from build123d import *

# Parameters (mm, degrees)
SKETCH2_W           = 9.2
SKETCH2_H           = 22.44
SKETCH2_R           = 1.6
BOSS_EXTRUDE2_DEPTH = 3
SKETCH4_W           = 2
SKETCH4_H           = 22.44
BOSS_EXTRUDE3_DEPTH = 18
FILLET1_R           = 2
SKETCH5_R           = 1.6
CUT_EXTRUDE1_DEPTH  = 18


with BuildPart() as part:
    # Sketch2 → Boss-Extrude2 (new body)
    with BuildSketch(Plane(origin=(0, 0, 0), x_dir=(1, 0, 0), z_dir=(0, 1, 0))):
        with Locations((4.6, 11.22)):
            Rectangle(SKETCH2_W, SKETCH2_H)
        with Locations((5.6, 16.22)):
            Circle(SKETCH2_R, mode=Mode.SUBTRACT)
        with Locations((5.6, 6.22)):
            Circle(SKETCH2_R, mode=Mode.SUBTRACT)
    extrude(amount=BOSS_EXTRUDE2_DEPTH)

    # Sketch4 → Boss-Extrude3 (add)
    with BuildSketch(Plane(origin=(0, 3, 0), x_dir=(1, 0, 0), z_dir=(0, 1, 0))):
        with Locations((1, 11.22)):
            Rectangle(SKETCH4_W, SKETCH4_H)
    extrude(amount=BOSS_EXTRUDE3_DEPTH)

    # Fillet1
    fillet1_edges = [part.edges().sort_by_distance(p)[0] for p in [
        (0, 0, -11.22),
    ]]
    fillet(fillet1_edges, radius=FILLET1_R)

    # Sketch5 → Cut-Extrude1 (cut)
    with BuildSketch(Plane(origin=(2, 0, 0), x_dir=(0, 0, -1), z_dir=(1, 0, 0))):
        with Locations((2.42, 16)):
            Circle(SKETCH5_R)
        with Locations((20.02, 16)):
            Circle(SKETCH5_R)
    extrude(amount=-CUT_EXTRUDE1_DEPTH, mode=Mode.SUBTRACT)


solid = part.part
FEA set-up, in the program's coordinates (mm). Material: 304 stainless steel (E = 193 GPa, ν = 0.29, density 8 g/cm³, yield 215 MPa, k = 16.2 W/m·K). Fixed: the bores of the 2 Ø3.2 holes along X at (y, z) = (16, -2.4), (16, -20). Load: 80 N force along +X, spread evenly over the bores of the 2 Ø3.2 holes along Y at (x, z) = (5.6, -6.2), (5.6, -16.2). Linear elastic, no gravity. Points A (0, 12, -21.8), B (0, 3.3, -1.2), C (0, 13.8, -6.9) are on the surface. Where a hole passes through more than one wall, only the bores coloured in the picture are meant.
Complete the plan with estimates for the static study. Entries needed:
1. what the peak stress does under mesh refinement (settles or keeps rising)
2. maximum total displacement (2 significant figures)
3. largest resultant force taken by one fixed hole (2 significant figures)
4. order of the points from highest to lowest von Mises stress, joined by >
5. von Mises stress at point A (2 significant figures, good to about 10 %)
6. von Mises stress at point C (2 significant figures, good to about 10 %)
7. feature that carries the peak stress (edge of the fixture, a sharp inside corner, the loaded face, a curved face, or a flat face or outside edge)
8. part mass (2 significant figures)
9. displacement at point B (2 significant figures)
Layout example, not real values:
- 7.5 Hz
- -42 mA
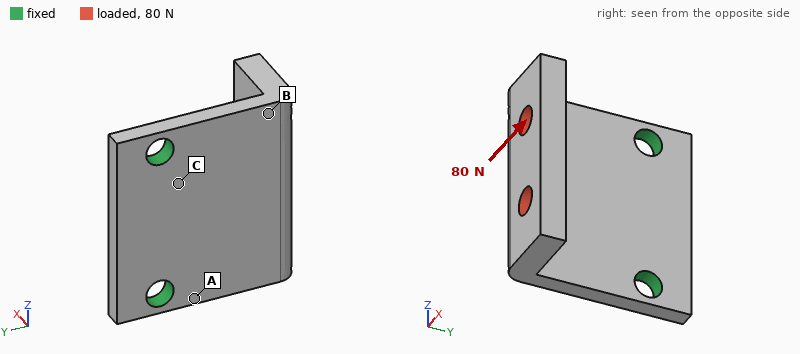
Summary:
- keeps rising
- 38 µm
- 40 N
- A > C > B
- 72 MPa
- 44 MPa
- edge of the fixture
- 11 g
- 22 µm
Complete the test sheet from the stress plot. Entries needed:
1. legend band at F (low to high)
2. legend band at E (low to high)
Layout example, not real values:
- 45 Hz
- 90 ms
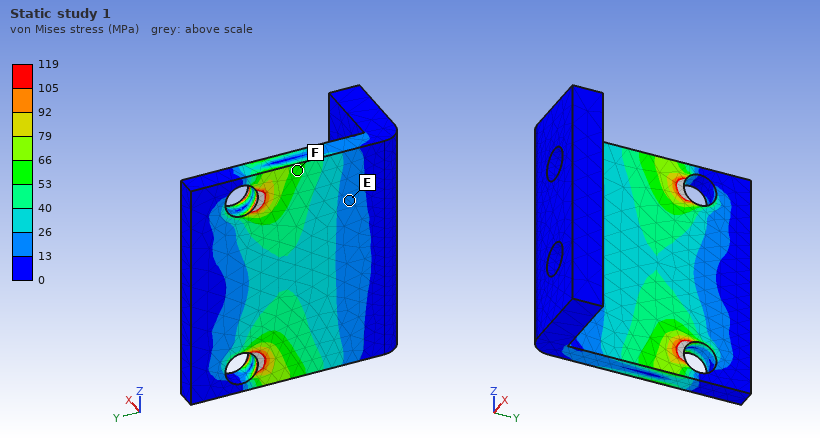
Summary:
- 53 to 66 MPa
- 13 to 26 MPa
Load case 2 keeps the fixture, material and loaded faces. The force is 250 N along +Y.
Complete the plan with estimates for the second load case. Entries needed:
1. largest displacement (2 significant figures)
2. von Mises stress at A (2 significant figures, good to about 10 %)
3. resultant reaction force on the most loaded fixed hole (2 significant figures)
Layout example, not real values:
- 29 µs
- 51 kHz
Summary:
- 65 µm
- 86 MPa
- 130 N
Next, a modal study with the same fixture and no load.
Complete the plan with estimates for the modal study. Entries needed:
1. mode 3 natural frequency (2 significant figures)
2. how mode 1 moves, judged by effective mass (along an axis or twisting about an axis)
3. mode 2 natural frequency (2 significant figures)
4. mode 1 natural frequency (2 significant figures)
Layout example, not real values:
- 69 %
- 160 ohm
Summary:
- 14 kHz
- along X
- 7700 Hz
- 3500 Hz
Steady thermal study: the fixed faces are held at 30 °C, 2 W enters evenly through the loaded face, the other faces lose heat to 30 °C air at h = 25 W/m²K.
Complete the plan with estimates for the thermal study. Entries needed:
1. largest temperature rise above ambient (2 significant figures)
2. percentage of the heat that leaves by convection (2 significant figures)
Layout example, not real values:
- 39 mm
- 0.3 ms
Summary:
- 39 K
- 32 %
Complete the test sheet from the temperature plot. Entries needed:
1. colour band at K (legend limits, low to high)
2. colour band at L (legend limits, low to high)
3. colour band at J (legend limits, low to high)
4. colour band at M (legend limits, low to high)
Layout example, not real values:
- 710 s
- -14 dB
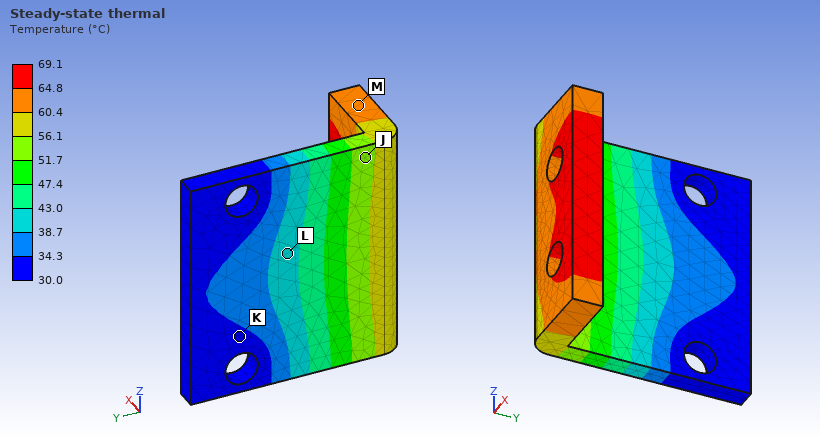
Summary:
- 30.0 to 34.3 °C
- 38.7 to 43.0 °C
- 51.7 to 56.1 °C
- 60.4 to 64.8 °C
